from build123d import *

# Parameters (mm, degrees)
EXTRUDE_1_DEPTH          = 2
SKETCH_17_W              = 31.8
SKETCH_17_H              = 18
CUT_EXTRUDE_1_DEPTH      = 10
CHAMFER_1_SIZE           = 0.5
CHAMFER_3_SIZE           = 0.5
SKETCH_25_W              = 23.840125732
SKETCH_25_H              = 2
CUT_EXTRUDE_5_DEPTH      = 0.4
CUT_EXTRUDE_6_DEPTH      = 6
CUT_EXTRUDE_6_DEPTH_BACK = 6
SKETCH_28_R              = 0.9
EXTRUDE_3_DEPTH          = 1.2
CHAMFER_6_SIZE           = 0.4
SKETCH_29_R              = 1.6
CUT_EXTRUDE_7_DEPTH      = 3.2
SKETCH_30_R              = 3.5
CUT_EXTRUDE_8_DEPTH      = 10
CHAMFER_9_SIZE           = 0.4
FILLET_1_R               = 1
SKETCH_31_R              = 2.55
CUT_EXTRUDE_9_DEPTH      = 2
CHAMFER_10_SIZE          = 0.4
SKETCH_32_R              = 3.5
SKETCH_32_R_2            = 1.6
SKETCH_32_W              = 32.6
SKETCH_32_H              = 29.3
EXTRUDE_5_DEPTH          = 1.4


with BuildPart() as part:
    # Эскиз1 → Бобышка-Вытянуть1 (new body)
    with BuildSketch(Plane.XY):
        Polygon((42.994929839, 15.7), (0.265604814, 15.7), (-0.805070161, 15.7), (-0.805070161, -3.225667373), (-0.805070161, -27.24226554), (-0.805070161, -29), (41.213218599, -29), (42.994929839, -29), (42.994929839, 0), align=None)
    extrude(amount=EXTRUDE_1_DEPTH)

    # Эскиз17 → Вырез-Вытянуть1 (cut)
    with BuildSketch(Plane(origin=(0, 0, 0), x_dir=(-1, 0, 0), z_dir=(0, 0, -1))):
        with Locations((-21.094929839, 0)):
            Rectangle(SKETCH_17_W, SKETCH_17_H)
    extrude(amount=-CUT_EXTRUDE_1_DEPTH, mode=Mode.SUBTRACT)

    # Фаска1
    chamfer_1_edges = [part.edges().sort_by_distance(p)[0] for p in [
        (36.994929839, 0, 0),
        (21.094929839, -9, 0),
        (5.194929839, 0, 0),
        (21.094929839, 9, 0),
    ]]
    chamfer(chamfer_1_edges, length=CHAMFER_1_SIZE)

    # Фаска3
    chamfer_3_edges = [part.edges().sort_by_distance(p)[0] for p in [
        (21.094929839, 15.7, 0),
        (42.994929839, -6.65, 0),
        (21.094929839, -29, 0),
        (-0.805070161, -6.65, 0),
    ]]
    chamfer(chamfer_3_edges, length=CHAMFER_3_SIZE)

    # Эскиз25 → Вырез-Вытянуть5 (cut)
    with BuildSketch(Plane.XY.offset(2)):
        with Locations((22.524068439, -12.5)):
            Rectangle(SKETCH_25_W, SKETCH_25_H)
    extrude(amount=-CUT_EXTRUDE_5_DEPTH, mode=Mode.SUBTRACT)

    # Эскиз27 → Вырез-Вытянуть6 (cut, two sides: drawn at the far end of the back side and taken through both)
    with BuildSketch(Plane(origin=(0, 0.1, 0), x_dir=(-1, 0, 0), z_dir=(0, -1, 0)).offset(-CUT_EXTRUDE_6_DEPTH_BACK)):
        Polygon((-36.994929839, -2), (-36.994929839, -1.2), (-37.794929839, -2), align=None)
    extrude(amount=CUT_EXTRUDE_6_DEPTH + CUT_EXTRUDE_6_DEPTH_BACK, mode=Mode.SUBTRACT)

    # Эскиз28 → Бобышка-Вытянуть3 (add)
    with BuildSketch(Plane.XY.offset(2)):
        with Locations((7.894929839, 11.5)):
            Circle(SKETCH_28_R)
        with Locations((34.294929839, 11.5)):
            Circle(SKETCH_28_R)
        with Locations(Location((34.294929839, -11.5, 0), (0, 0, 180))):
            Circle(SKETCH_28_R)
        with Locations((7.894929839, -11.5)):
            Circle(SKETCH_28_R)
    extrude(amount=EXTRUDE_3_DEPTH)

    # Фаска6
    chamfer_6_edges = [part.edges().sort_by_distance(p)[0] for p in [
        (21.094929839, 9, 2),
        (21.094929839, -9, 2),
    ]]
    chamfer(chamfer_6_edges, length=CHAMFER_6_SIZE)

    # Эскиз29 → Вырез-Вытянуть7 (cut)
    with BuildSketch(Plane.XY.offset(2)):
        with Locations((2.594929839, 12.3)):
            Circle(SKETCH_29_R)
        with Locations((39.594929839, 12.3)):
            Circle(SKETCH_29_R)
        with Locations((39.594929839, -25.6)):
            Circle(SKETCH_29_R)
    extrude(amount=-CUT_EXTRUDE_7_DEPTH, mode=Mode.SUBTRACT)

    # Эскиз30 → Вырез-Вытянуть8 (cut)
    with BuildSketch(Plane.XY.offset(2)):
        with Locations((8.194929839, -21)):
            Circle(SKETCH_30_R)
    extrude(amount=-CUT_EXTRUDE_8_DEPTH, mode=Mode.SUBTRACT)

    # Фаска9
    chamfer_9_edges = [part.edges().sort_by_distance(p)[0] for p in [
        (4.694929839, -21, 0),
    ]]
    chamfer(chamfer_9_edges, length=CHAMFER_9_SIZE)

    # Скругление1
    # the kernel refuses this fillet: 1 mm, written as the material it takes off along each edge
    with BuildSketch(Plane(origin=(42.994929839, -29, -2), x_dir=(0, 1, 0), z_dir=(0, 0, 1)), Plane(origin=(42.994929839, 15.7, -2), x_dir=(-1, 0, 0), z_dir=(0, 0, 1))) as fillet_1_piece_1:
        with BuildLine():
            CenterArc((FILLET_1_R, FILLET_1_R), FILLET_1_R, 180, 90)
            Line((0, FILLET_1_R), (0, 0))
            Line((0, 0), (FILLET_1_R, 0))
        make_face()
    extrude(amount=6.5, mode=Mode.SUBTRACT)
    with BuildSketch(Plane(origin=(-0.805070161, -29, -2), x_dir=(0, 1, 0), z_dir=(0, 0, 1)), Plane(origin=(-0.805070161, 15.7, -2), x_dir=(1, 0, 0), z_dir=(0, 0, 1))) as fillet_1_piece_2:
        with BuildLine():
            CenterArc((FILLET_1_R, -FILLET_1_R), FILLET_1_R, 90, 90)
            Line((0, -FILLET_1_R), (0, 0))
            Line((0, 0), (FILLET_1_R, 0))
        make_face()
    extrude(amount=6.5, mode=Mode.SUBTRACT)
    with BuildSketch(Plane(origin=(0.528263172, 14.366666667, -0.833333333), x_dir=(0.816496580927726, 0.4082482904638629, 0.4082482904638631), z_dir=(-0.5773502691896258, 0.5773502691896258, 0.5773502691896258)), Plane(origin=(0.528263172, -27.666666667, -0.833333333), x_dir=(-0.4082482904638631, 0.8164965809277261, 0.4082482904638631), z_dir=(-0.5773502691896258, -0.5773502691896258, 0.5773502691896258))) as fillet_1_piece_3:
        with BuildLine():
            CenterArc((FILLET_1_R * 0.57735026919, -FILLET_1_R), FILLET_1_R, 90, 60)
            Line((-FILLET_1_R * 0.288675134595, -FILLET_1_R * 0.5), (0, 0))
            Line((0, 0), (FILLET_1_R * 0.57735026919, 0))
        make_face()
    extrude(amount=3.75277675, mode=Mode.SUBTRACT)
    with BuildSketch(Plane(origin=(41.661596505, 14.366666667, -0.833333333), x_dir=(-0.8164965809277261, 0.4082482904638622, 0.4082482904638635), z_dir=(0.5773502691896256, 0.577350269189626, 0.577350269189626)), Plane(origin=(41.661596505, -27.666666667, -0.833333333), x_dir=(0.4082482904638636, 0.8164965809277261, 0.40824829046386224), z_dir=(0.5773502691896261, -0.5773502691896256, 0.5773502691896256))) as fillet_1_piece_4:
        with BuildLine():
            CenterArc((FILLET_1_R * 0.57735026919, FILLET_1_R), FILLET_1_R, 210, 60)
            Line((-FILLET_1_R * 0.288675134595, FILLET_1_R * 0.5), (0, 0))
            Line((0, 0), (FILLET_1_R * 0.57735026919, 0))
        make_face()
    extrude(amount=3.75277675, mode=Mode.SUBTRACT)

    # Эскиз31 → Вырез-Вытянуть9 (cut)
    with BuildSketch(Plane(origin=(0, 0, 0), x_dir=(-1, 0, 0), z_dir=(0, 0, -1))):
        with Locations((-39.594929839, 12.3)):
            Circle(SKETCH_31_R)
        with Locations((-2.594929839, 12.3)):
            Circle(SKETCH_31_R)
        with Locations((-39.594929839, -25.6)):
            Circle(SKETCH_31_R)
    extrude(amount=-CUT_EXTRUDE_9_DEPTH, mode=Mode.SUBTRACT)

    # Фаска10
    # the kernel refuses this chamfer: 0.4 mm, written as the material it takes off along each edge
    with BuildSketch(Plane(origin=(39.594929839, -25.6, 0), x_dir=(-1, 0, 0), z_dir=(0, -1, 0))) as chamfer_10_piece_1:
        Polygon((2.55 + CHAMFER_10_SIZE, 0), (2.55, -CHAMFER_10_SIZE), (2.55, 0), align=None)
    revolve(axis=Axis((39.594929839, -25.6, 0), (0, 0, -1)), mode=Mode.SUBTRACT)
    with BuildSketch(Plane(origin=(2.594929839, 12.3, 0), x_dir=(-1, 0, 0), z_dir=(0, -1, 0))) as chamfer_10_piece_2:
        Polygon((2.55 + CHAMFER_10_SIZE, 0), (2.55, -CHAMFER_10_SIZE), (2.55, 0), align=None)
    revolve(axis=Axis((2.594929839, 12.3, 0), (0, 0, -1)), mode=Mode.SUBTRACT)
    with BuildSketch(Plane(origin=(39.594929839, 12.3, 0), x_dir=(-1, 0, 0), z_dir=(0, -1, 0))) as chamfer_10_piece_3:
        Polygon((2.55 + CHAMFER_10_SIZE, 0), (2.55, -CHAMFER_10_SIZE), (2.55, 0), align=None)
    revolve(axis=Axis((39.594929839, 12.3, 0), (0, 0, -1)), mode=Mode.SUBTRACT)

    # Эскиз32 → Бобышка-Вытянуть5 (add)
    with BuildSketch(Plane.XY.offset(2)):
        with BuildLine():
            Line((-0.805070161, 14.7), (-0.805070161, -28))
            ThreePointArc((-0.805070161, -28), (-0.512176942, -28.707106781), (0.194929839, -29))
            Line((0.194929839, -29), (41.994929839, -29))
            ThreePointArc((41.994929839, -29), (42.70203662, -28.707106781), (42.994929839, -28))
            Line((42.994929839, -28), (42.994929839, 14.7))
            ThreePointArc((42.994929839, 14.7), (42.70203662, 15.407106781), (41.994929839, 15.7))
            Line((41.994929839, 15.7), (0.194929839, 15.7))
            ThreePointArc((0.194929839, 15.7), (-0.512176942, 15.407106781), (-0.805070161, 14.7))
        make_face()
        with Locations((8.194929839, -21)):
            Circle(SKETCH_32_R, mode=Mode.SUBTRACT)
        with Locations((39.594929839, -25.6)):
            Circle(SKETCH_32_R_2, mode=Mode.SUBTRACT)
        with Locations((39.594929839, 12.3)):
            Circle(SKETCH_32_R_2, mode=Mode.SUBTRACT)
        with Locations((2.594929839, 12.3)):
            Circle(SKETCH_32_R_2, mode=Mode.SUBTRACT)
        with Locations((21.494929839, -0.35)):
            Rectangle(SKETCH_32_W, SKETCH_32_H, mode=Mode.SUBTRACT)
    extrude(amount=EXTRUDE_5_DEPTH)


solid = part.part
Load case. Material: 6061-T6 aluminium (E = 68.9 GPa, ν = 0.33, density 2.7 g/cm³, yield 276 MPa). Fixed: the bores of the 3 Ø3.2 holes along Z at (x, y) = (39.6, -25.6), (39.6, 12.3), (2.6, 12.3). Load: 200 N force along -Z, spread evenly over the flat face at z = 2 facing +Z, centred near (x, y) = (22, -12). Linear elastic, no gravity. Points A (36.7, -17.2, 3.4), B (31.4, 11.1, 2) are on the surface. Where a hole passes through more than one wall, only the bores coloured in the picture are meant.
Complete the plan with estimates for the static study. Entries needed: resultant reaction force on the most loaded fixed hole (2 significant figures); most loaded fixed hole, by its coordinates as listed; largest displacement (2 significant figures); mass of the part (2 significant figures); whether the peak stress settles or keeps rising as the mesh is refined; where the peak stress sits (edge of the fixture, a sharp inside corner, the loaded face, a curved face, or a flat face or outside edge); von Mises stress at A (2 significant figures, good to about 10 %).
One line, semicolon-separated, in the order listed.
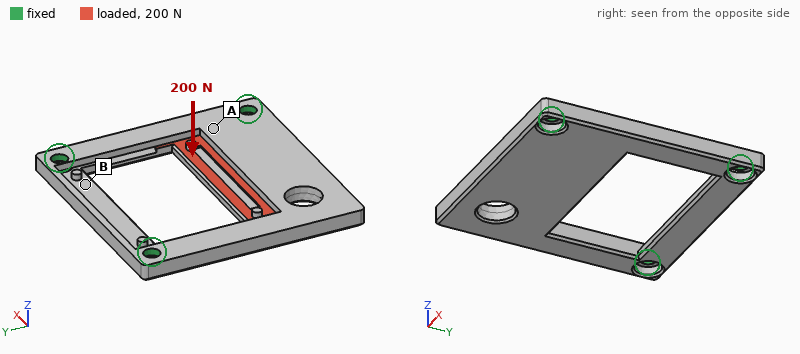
160 N; (39.6, -25.6); 0.17 mm; 10 g; keeps rising; edge of the fixture; 23 MPa
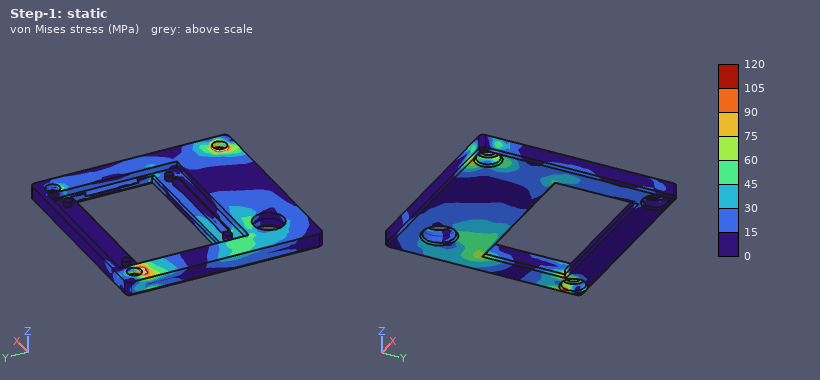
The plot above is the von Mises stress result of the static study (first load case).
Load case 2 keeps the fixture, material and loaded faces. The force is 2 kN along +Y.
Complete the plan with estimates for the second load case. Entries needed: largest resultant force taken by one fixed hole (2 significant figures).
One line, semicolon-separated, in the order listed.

910 N
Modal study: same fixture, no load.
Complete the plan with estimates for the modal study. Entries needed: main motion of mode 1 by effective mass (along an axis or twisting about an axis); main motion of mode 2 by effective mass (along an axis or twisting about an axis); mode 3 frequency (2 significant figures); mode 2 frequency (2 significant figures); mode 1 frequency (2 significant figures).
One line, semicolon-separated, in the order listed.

along Z; along Z; 8300 Hz; 6900 Hz; 2100 Hz
